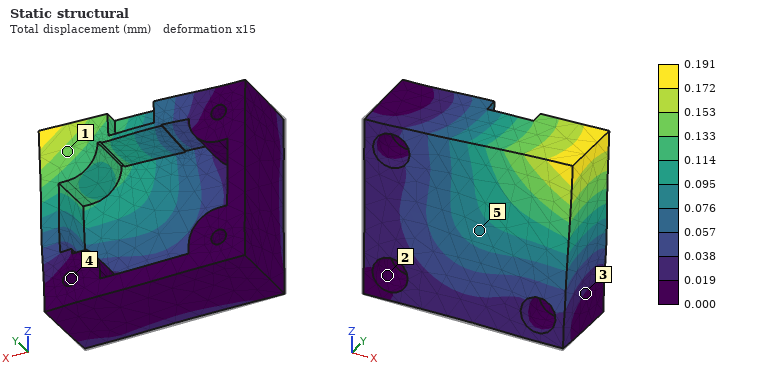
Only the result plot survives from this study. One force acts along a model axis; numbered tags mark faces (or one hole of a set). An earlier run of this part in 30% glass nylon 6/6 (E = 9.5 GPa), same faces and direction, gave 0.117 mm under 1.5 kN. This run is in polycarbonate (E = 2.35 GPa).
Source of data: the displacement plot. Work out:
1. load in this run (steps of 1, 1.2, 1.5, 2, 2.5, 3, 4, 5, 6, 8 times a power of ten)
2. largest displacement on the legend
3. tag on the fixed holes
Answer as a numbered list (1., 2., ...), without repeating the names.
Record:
1. 600 N
2. 0.191 mm
3. 4
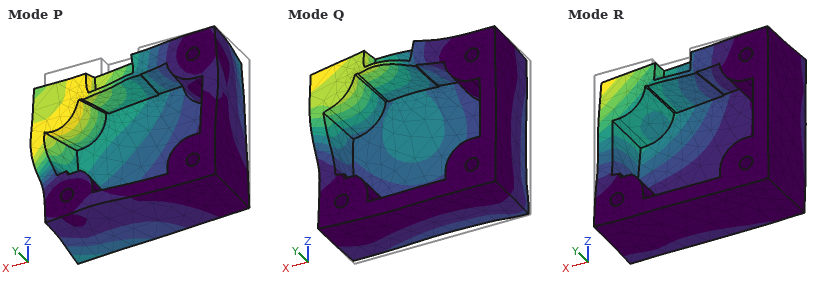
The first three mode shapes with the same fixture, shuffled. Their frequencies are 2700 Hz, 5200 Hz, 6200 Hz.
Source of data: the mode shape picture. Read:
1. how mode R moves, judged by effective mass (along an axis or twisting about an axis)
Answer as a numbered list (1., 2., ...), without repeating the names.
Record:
1. along Y
